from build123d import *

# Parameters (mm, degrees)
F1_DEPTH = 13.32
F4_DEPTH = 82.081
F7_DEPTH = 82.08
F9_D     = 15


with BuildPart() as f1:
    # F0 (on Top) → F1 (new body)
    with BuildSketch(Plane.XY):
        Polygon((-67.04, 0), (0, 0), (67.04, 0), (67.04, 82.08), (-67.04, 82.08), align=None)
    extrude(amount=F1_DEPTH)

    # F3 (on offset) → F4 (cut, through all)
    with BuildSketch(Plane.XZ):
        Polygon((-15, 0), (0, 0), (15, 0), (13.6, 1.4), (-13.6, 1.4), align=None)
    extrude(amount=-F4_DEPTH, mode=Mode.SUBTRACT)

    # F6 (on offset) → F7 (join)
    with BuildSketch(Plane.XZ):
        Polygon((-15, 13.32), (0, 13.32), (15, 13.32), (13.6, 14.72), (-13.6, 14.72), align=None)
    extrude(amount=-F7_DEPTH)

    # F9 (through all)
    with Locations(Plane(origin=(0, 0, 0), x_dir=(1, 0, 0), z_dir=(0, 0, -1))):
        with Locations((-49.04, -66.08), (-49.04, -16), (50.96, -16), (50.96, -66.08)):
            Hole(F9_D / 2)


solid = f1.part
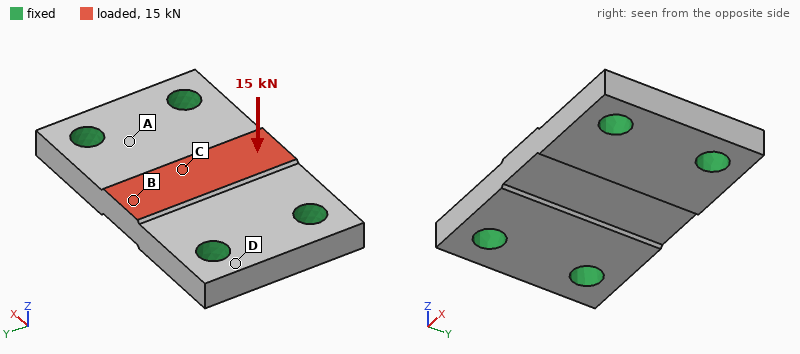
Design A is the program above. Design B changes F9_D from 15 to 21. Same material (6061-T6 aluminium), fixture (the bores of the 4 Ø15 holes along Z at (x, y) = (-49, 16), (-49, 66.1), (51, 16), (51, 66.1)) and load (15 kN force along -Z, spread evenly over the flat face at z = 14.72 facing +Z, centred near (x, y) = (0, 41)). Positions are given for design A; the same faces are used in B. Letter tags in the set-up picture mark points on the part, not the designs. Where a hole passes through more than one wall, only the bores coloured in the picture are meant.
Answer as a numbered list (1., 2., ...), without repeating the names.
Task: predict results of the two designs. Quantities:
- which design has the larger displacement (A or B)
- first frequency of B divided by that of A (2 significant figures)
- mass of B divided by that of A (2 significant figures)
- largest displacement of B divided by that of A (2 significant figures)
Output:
1. A
2. 1.2
3. 0.93
4. 0.79
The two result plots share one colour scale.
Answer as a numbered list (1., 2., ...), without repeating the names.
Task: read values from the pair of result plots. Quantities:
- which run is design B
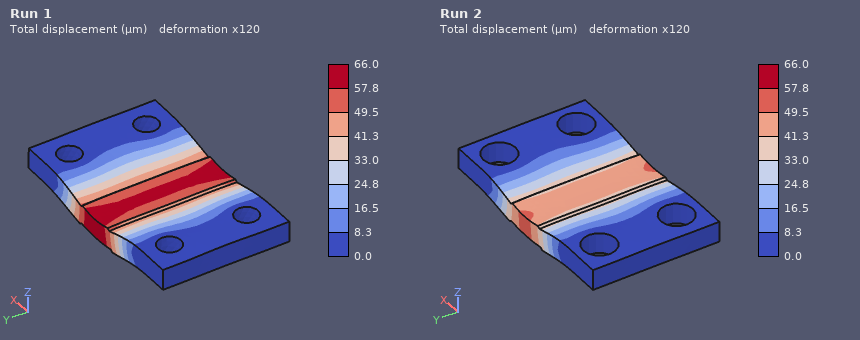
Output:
1. Run 2
